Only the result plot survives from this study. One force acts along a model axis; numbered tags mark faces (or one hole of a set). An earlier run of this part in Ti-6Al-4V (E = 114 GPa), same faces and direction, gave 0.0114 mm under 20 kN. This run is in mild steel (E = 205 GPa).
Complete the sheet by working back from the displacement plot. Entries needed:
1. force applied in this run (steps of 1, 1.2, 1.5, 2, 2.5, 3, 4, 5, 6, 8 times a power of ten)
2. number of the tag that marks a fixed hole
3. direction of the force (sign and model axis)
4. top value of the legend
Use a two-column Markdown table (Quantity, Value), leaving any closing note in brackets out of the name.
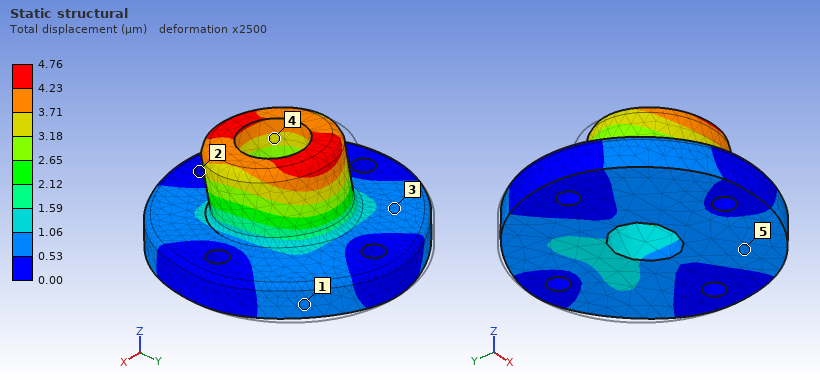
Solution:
| Quantity | Value |
|---|---|
| force applied in this run | 15 kN |
| number of the tag that marks a fixed hole | 2 |
| direction of the force | -Y |
| top value of the legend | 4.76 µm |
